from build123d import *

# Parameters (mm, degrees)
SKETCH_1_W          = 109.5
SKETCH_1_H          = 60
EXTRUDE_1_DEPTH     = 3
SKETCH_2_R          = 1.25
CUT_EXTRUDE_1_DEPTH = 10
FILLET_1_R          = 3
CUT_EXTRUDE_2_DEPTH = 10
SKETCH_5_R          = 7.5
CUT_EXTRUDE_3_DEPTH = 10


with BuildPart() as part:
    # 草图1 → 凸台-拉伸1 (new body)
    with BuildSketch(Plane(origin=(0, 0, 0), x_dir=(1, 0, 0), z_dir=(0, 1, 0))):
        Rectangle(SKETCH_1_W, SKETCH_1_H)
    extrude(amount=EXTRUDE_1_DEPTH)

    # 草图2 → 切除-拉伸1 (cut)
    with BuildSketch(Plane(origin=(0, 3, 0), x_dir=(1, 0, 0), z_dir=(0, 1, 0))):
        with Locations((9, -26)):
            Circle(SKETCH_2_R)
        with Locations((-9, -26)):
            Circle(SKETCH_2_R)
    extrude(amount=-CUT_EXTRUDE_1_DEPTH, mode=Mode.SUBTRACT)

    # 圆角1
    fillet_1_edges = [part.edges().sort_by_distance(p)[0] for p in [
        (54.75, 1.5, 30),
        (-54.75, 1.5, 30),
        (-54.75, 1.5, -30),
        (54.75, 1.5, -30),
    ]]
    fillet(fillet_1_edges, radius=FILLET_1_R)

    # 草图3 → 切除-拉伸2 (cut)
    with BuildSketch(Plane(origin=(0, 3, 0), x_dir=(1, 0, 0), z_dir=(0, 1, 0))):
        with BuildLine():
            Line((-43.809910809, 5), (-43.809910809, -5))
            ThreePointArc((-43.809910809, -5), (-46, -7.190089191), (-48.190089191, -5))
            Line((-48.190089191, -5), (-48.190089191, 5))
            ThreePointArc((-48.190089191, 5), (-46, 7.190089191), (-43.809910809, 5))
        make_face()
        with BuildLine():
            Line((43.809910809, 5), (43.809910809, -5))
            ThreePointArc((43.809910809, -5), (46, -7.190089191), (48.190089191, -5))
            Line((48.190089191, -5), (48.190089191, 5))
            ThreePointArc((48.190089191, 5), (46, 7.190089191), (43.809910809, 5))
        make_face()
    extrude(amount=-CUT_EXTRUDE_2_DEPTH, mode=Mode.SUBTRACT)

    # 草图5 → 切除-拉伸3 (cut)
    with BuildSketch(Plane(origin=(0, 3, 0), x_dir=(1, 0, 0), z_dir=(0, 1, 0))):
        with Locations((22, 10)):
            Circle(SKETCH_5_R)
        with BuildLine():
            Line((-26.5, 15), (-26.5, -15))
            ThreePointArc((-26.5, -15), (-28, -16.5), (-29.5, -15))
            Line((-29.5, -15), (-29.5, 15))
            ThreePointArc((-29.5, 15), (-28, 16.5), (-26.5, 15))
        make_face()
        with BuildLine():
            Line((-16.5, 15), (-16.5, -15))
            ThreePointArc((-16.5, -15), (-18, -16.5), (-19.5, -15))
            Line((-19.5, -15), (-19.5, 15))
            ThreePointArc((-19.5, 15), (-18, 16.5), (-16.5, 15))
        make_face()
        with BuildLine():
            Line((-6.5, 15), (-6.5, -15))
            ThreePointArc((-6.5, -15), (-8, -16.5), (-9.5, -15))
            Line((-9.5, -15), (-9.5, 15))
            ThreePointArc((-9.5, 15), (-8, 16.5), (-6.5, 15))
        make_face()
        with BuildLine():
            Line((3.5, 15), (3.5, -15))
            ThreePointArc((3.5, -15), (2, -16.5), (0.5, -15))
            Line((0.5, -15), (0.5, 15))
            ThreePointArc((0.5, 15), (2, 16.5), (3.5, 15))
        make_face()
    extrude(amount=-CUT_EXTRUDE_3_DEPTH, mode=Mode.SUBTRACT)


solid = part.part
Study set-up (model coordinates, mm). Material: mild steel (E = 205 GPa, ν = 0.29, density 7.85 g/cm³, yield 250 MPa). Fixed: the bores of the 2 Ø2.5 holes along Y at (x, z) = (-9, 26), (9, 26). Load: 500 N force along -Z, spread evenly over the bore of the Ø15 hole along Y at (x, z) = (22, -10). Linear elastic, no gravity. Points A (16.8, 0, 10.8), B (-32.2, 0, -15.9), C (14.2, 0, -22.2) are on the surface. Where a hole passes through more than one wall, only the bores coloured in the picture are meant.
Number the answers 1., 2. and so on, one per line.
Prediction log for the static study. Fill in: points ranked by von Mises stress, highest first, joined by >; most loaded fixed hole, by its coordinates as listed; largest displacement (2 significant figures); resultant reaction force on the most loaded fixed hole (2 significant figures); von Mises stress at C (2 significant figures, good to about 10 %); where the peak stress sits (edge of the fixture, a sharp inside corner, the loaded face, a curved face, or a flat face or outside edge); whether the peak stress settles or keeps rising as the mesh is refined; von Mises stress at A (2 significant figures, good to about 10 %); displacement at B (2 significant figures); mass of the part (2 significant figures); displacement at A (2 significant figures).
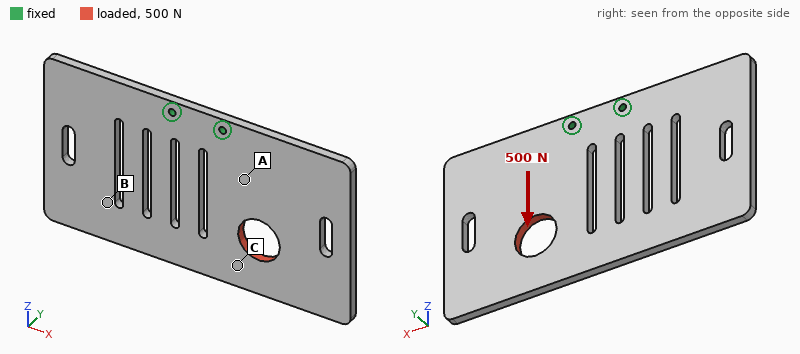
1. A > C > B
2. (9, 26)
3. 16 µm
4. 800 N
5. 4.7 MPa
6. edge of the fixture
7. keeps rising
8. 8.9 MPa
9. 9.4 µm
10. 140 g
11. 4.3 µm
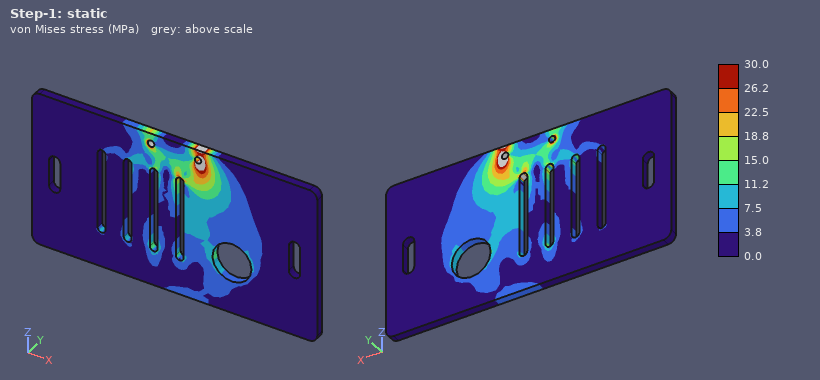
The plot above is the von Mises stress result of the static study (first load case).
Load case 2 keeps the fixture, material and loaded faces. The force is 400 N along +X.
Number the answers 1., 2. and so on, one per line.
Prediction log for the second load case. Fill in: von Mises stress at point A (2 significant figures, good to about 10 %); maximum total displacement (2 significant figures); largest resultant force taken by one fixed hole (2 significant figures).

1. 11 MPa
2. 27 µm
3. 740 N
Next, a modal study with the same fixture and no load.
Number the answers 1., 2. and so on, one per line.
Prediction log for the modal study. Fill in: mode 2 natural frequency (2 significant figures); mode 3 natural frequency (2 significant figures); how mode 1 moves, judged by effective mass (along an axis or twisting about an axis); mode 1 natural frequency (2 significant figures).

1. 550 Hz
2. 1000 Hz
3. along Y
4. 480 Hz
